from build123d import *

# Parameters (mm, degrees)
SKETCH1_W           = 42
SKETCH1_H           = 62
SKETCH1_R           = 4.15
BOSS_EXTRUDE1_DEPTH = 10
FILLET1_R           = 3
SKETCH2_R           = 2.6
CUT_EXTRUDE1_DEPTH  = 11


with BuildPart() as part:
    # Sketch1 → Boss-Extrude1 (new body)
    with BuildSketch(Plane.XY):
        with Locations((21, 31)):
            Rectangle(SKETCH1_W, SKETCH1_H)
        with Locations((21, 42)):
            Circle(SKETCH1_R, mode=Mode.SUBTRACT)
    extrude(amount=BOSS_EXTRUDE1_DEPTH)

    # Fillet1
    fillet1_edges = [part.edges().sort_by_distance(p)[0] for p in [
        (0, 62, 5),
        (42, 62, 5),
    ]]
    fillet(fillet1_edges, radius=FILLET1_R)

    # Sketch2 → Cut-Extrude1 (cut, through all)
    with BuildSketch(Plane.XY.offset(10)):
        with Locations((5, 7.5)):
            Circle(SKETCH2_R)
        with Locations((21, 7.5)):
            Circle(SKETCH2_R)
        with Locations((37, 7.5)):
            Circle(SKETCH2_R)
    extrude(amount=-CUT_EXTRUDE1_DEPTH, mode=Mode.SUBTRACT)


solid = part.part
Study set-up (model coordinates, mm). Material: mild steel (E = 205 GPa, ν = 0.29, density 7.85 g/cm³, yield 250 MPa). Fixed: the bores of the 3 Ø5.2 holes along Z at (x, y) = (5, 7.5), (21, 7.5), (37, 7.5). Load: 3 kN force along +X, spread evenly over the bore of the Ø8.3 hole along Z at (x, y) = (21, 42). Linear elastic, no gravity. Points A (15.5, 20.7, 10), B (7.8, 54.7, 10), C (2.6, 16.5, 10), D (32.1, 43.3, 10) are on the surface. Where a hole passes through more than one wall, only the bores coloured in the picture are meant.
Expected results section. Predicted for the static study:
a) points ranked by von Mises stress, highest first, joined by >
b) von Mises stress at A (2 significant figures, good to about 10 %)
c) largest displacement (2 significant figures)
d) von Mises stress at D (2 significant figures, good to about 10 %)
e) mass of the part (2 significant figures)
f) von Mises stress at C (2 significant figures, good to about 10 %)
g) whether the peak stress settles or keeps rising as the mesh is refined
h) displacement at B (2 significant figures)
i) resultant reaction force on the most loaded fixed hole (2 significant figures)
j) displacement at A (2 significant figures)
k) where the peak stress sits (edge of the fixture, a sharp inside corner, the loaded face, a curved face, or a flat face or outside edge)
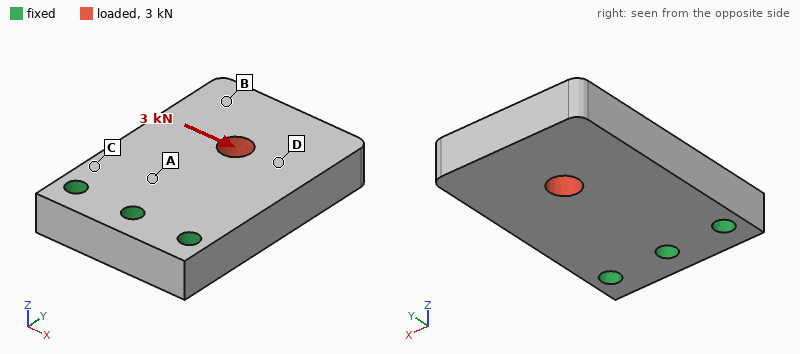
C > A > D > B
17 MPa
10.0 µm
9.7 MPa
190 g
24 MPa
keeps rising
8.8 µm
3.1 kN
1.7 µm
edge of the fixture
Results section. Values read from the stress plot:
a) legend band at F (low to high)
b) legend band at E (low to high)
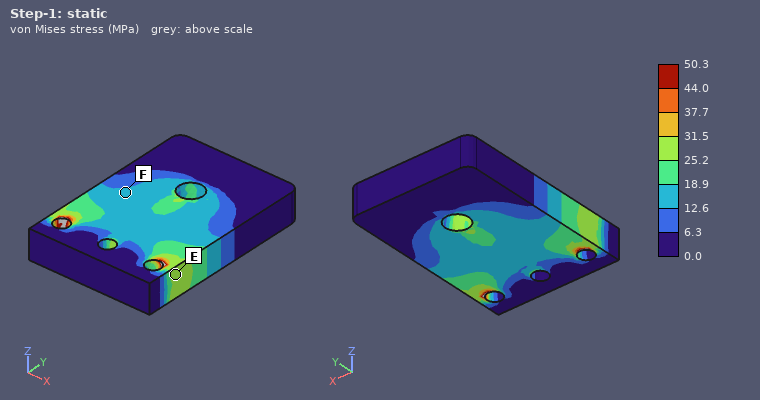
12.6 to 18.9 MPa
25.2 to 31.5 MPa
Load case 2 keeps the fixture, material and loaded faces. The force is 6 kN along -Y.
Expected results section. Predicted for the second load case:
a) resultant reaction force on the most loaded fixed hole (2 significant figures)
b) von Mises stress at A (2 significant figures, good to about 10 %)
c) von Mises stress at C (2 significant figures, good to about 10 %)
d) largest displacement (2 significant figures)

2.1 kN
15 MPa
14 MPa
3.8 µm
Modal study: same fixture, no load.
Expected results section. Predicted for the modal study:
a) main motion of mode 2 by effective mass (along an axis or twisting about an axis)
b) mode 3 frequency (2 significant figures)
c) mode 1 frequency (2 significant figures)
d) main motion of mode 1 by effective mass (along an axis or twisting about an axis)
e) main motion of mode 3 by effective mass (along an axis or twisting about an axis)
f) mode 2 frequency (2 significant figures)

twisting about Y
8800 Hz
2800 Hz
along Z
along X
7400 Hz
